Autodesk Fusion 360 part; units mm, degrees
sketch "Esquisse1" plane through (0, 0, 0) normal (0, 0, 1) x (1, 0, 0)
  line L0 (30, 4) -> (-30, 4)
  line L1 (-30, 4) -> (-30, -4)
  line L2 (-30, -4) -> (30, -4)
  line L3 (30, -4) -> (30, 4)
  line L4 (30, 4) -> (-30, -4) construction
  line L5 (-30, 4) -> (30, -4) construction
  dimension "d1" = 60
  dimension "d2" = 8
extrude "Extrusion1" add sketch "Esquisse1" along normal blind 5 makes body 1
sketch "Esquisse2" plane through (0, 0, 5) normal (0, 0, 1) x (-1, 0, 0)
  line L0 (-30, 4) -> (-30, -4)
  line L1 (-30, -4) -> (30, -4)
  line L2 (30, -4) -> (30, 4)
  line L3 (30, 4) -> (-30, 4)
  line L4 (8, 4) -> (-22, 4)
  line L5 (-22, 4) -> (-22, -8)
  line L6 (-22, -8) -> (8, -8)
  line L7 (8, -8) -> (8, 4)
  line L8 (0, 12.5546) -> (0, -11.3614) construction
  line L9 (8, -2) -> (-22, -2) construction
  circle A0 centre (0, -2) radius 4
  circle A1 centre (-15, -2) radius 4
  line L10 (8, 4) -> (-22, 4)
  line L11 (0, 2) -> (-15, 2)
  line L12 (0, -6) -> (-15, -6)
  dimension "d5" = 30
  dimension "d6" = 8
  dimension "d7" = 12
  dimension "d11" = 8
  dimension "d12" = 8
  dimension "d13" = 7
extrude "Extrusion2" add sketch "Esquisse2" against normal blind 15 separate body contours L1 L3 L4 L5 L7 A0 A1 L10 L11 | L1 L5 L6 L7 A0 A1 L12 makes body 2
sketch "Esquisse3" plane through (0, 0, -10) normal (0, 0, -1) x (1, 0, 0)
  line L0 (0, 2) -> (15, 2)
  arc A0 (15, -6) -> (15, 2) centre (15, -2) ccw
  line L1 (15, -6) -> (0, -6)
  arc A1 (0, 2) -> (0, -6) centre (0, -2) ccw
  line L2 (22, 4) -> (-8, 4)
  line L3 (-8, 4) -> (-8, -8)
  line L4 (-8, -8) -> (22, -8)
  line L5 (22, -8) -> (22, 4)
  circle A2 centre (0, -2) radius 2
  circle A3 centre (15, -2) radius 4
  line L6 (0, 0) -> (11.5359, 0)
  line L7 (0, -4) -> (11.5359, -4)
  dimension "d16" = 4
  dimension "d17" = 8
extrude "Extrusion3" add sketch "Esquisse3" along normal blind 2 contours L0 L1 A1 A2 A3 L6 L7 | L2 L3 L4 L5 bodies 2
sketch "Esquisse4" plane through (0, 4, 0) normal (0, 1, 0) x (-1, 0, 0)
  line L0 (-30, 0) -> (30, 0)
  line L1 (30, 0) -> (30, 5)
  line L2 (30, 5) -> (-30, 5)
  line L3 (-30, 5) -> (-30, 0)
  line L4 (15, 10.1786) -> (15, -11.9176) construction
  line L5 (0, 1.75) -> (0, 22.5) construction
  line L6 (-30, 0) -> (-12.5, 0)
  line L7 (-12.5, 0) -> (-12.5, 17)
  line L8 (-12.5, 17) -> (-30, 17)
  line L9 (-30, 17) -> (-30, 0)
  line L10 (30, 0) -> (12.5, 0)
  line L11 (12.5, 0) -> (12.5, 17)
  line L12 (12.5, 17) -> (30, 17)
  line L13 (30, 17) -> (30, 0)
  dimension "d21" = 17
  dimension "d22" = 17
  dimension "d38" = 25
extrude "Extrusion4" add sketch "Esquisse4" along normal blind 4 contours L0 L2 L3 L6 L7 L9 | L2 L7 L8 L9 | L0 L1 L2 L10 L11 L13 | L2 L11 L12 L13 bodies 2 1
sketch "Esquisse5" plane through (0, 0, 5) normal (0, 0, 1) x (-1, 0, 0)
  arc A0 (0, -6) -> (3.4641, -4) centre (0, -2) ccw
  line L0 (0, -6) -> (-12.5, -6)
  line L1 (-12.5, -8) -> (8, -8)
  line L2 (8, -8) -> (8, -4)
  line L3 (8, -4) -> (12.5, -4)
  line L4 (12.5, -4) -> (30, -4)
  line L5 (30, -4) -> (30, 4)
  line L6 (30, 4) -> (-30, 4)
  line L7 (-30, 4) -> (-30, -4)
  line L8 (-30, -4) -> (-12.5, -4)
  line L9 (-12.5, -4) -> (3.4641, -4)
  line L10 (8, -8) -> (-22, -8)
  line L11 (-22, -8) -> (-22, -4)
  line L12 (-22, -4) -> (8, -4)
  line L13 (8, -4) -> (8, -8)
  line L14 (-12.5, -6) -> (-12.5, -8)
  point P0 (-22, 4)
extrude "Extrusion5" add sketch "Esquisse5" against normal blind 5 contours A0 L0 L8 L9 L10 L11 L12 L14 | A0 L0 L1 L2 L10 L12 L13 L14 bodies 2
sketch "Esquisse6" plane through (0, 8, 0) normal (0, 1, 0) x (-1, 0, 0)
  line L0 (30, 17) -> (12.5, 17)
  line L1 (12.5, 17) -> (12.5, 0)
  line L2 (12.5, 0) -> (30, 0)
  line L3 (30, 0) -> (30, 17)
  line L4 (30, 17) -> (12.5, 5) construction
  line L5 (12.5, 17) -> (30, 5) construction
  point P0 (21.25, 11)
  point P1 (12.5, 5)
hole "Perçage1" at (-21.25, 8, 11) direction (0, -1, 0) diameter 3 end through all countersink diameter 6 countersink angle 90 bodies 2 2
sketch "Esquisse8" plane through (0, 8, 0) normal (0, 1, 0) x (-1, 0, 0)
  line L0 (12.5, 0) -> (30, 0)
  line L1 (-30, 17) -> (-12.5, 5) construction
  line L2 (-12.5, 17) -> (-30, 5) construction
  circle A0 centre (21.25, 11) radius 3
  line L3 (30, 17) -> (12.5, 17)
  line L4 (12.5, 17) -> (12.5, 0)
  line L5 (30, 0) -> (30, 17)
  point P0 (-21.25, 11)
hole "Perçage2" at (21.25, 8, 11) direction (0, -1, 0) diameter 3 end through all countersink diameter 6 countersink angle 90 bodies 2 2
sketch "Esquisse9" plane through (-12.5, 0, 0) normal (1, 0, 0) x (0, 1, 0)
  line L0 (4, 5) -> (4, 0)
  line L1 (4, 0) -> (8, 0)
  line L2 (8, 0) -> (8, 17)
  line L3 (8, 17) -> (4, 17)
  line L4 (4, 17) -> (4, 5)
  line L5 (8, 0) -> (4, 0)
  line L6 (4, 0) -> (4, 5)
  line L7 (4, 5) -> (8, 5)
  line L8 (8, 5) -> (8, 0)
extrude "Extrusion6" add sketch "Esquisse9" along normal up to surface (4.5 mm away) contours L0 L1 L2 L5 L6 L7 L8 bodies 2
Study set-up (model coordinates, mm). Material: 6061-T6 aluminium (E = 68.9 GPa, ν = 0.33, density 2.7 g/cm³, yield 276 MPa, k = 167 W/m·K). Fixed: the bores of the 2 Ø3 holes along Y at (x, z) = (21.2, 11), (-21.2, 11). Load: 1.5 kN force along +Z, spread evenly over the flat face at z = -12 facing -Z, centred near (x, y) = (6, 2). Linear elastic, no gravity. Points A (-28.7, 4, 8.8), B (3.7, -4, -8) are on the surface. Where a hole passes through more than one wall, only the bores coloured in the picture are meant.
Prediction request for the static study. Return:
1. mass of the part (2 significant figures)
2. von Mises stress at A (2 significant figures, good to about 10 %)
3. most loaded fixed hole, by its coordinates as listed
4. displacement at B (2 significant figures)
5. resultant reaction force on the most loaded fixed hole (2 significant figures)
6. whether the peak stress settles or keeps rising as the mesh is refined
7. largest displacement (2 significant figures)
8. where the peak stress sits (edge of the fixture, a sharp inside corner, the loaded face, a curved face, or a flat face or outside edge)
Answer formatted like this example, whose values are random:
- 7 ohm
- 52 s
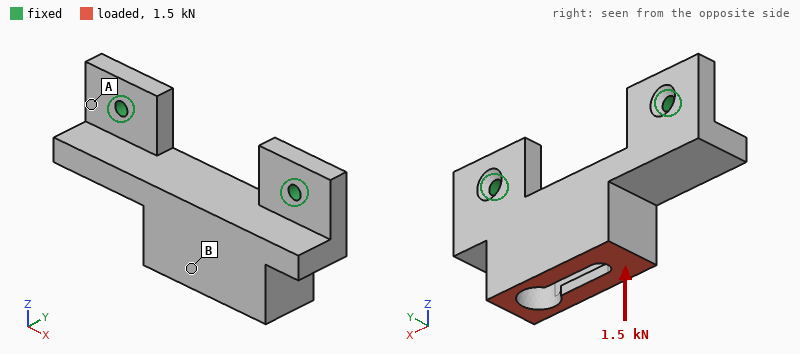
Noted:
- 21 g
- 32 MPa
- (21.2, 11)
- 0.12 mm
- 1.0 kN
- keeps rising
- 0.14 mm
- edge of the fixture
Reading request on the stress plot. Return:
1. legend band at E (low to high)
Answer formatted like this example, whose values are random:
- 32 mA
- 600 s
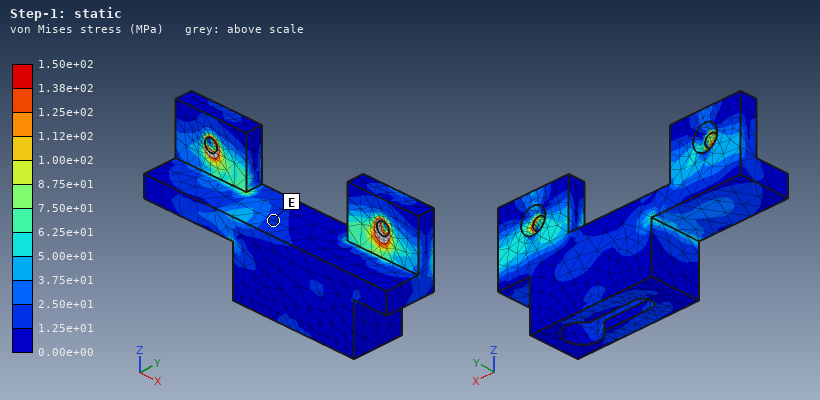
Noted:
- 1.25e+01 to 2.50e+01 MPa
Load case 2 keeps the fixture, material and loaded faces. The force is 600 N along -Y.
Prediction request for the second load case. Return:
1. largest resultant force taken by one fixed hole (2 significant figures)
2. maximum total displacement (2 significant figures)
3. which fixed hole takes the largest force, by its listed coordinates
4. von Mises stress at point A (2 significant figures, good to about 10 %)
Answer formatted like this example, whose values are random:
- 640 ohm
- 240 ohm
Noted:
- 390 N
- 0.32 mm
- (21.2, 11)
- 70 MPa
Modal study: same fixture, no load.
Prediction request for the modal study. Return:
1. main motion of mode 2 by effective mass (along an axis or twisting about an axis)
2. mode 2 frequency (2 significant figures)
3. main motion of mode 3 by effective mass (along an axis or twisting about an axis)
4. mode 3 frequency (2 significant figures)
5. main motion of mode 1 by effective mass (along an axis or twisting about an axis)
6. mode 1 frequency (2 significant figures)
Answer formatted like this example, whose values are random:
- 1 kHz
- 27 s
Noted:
- twisting about Z
- 9600 Hz
- along X
- 13 kHz
- along Y
- 3200 Hz
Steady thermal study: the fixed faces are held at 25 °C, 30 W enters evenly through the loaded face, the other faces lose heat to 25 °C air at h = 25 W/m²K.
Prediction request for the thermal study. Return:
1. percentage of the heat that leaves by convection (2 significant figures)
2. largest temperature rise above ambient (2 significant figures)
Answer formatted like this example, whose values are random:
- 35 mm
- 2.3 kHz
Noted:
- 7.0 %
- 36 K
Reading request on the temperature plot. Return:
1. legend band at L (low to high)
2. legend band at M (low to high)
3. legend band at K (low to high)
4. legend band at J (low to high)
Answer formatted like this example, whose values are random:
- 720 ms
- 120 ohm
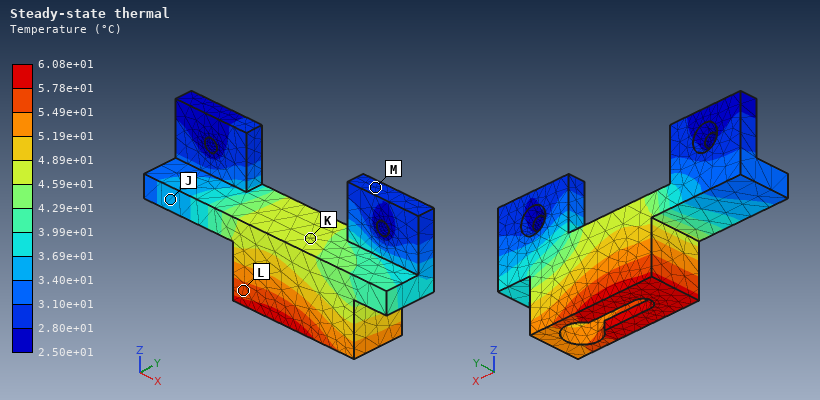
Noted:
- 5.49e+01 to 5.78e+01 °C
- 2.80e+01 to 3.10e+01 °C
- 4.59e+01 to 4.89e+01 °C
- 3.40e+01 to 3.69e+01 °C
